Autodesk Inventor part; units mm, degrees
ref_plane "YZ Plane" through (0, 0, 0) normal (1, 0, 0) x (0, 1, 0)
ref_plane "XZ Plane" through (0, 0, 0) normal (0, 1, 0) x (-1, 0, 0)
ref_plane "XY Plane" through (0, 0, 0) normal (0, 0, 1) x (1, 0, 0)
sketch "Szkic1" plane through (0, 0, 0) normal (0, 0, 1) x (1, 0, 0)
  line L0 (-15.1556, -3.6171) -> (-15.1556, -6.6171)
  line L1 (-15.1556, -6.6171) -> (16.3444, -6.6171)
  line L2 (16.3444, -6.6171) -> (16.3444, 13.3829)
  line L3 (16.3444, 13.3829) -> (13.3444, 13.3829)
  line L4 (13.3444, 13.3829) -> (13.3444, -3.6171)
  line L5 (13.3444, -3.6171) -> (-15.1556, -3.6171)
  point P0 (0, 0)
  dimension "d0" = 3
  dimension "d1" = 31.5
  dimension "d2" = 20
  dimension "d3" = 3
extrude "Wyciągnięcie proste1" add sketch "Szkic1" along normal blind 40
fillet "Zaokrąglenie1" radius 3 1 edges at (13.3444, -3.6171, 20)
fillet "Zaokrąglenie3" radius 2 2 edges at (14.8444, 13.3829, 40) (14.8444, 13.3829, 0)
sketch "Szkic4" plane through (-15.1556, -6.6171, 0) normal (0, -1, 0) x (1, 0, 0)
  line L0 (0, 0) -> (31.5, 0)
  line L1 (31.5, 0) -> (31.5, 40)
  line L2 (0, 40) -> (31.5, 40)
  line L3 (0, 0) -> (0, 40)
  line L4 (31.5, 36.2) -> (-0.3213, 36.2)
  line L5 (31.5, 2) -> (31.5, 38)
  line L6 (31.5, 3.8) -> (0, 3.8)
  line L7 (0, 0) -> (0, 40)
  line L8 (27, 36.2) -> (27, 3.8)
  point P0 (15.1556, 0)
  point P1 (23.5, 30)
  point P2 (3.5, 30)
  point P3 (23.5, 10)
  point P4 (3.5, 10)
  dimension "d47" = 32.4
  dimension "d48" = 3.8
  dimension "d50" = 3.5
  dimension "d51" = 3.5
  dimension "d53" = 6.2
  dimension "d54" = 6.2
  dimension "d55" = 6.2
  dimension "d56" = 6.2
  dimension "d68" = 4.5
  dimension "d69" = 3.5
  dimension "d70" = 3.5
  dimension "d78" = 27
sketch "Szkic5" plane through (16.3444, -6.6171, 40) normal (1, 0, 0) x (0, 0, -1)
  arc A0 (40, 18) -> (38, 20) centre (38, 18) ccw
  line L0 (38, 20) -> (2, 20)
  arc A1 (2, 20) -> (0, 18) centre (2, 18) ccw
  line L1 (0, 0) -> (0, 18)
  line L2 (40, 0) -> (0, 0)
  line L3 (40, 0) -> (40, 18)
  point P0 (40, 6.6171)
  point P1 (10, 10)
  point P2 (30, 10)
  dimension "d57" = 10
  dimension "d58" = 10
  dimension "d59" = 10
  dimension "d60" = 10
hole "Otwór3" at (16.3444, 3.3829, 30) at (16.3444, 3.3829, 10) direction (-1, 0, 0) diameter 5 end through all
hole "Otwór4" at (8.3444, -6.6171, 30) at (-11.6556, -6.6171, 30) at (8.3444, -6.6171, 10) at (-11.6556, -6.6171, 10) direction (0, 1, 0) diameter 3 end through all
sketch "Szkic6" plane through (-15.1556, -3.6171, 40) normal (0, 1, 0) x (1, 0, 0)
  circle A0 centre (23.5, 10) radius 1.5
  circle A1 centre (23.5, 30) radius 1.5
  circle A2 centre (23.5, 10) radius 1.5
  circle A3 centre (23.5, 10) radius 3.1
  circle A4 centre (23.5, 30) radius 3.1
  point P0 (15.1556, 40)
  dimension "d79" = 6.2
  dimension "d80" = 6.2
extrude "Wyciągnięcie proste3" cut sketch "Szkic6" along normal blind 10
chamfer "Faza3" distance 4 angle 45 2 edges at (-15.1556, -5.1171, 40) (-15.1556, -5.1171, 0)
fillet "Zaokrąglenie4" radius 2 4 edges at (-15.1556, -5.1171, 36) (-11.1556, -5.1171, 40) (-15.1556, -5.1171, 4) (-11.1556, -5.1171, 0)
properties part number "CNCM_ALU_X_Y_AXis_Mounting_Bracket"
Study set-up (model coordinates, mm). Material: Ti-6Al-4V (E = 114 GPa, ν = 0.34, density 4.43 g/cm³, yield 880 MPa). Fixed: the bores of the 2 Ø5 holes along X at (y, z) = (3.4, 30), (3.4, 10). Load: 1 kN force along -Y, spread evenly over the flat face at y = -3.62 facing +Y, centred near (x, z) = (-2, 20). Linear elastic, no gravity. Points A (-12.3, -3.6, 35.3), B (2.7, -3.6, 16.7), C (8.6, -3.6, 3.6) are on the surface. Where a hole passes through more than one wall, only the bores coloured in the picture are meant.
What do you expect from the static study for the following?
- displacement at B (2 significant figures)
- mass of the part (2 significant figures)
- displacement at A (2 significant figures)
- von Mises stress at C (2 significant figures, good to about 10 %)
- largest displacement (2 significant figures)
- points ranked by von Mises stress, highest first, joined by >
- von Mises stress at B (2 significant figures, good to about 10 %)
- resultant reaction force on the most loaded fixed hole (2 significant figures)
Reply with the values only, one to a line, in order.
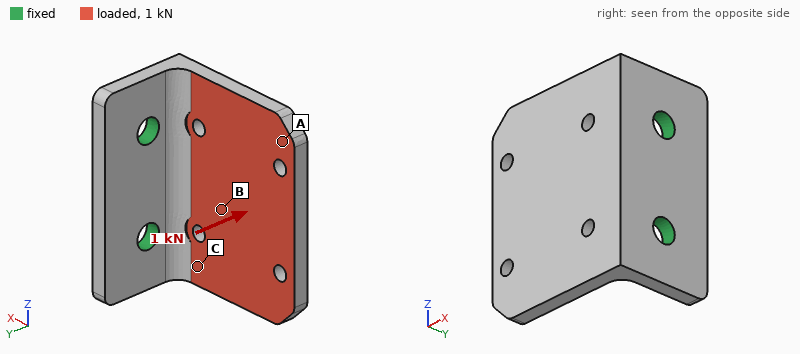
0.17 mm
25 g
0.49 mm
180 MPa
0.56 mm
C > B > A
95 MPa
510 N
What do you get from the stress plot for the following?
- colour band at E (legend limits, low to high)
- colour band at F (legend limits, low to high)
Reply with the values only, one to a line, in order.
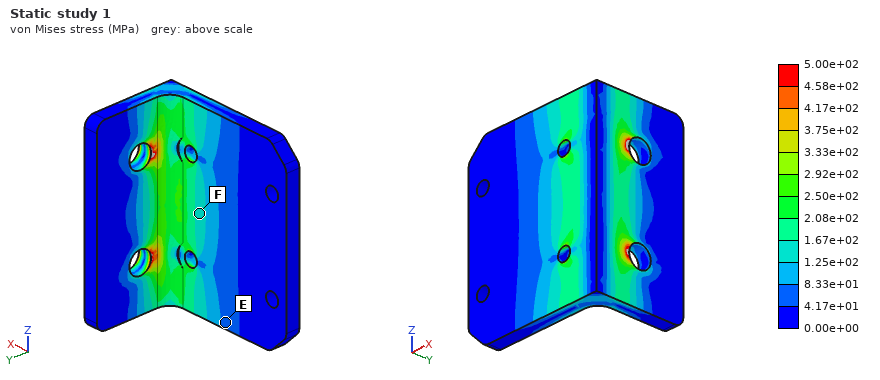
4.17e+01 to 8.33e+01 MPa
1.25e+02 to 1.67e+02 MPa
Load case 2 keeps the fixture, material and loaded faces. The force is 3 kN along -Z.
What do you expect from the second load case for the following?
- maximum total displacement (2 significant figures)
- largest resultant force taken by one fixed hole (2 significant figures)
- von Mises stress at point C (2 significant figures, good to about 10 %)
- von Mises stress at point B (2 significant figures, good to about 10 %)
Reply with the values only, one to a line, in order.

0.23 mm
2.7 kN
150 MPa
110 MPa
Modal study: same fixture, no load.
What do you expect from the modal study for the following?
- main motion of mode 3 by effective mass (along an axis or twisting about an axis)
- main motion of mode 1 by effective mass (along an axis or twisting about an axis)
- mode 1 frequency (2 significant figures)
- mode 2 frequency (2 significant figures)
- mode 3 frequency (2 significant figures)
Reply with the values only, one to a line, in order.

along Z
along Y
2300 Hz
4800 Hz
7700 Hz
